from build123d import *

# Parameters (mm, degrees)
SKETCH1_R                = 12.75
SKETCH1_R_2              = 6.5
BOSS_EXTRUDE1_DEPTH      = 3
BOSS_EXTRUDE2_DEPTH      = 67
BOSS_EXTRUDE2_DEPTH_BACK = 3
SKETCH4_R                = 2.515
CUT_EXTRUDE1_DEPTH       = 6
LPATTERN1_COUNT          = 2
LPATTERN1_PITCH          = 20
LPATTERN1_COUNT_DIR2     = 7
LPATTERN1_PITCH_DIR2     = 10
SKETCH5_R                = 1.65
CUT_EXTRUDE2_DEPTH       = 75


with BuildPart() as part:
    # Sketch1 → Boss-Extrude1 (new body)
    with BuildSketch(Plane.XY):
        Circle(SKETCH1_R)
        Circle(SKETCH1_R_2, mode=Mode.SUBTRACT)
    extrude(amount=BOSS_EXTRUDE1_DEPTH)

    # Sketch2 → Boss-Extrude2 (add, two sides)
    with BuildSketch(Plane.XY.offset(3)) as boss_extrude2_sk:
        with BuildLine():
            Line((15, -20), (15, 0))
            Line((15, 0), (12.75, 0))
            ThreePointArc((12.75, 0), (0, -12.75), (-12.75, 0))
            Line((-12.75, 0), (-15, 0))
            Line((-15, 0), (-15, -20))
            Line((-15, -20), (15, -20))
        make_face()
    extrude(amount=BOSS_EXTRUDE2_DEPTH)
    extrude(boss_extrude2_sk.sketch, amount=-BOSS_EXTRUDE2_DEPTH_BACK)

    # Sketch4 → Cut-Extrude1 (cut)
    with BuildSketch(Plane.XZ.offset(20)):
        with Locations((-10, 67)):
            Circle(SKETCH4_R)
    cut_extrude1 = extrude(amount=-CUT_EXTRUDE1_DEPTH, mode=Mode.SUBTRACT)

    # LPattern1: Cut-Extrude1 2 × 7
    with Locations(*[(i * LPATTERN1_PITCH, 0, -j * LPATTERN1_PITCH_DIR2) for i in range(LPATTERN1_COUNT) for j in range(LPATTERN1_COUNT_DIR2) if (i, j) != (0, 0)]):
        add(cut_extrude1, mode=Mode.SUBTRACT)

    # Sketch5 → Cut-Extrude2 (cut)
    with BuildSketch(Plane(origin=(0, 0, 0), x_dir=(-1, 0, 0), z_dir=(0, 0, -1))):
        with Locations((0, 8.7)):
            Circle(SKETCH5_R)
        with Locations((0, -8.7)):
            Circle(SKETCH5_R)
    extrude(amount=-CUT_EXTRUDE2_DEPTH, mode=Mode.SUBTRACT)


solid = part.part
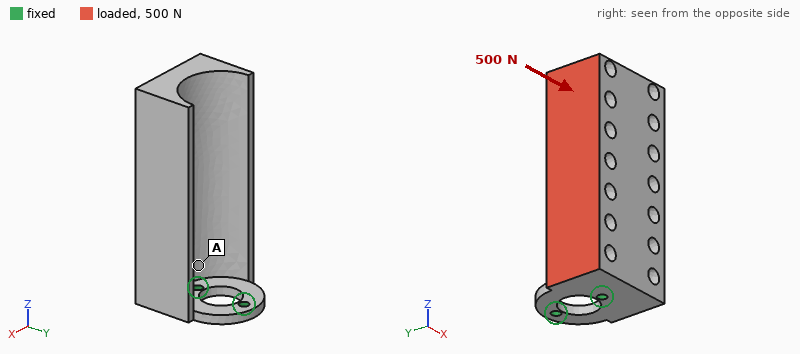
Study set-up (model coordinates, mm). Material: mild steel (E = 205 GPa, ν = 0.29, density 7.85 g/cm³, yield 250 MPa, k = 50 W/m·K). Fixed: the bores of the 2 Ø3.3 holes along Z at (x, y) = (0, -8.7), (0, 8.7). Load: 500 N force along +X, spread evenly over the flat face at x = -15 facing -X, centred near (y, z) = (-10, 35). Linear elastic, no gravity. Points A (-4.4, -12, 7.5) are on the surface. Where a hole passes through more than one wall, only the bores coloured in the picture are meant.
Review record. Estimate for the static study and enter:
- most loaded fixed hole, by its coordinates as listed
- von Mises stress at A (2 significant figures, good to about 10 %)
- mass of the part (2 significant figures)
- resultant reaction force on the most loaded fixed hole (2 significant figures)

(0, -8.7)
45 MPa
180 g
480 N
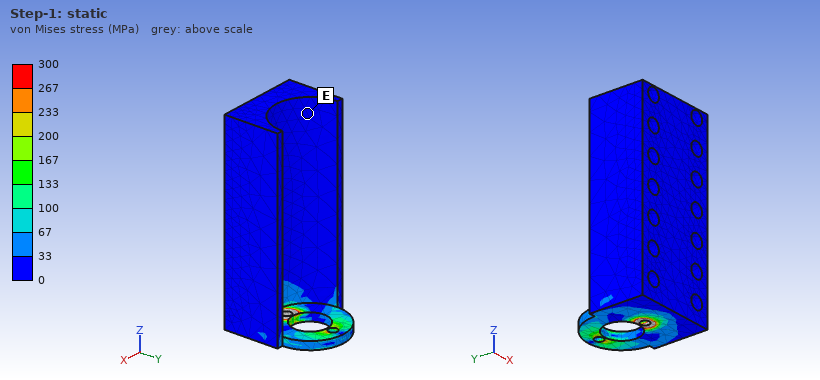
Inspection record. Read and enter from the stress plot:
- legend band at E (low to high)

0 to 33 MPa
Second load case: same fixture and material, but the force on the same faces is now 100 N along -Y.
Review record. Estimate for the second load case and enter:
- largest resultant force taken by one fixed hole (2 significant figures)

140 N
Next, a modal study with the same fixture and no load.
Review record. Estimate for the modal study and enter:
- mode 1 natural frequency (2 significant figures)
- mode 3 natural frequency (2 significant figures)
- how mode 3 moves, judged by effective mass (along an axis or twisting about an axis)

630 Hz
3900 Hz
twisting about Z
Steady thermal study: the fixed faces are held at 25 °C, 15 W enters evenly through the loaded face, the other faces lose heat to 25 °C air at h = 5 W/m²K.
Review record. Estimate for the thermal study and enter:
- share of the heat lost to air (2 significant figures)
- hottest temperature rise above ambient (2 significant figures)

12 %
59 K
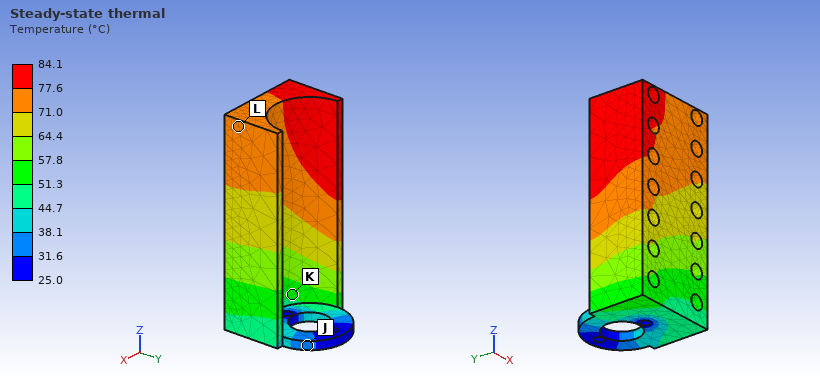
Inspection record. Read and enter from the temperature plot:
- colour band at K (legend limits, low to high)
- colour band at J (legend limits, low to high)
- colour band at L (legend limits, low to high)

51.3 to 57.8 °C
31.6 to 38.1 °C
71.0 to 77.6 °C
